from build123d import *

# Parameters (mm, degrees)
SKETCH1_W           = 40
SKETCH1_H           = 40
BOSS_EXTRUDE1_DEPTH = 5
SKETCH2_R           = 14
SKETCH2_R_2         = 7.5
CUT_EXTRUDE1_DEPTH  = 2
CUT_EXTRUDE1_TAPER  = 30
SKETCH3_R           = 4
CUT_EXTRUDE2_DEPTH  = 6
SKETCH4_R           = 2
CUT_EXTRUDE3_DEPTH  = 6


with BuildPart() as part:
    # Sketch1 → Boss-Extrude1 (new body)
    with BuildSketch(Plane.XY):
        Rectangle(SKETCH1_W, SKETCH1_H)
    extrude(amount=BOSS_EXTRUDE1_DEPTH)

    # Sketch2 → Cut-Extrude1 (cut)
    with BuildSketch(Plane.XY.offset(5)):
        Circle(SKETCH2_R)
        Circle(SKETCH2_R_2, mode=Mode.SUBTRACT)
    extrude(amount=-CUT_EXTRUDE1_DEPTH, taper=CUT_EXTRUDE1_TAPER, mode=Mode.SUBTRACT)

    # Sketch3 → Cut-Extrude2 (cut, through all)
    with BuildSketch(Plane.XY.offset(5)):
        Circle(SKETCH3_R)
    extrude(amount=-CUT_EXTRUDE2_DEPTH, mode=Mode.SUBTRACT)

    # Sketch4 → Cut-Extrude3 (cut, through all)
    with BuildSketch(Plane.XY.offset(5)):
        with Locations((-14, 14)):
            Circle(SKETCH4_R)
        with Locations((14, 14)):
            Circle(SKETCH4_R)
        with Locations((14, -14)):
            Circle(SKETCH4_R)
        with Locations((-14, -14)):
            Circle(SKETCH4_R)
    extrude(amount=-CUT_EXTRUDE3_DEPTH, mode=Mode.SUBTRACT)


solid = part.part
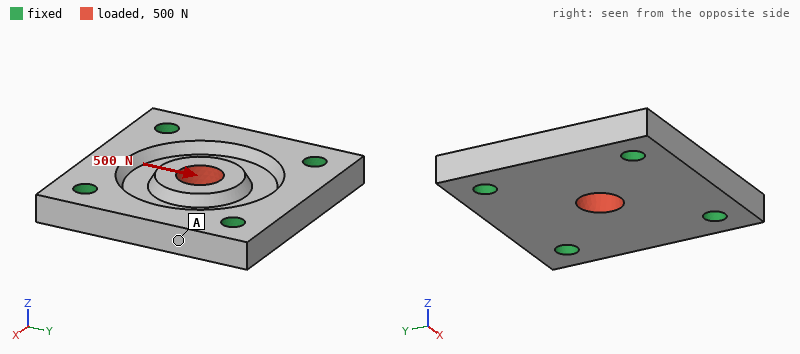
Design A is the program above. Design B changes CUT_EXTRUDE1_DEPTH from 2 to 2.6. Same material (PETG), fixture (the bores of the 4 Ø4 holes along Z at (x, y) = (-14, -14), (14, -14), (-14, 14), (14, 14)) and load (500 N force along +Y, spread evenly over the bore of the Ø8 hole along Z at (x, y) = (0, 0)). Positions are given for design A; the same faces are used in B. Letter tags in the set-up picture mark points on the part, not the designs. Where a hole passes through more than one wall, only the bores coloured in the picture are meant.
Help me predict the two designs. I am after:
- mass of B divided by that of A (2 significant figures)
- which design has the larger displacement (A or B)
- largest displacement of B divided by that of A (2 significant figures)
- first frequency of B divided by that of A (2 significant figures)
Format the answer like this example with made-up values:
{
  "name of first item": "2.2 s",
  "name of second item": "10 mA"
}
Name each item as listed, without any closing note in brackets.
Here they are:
{
  "mass of B divided by that of A": "0.98",
  "which design has the larger displacement": "B",
  "largest displacement of B divided by that of A": "1.2",
  "first frequency of B divided by that of A": "1.00"
}
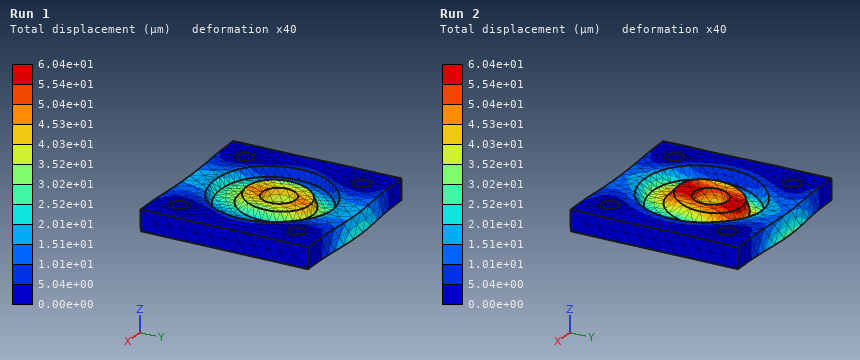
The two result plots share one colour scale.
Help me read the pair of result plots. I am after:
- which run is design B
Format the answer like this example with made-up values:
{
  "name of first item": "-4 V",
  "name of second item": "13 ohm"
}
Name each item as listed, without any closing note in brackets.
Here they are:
{
  "which run is design B": "Run 2"
}
